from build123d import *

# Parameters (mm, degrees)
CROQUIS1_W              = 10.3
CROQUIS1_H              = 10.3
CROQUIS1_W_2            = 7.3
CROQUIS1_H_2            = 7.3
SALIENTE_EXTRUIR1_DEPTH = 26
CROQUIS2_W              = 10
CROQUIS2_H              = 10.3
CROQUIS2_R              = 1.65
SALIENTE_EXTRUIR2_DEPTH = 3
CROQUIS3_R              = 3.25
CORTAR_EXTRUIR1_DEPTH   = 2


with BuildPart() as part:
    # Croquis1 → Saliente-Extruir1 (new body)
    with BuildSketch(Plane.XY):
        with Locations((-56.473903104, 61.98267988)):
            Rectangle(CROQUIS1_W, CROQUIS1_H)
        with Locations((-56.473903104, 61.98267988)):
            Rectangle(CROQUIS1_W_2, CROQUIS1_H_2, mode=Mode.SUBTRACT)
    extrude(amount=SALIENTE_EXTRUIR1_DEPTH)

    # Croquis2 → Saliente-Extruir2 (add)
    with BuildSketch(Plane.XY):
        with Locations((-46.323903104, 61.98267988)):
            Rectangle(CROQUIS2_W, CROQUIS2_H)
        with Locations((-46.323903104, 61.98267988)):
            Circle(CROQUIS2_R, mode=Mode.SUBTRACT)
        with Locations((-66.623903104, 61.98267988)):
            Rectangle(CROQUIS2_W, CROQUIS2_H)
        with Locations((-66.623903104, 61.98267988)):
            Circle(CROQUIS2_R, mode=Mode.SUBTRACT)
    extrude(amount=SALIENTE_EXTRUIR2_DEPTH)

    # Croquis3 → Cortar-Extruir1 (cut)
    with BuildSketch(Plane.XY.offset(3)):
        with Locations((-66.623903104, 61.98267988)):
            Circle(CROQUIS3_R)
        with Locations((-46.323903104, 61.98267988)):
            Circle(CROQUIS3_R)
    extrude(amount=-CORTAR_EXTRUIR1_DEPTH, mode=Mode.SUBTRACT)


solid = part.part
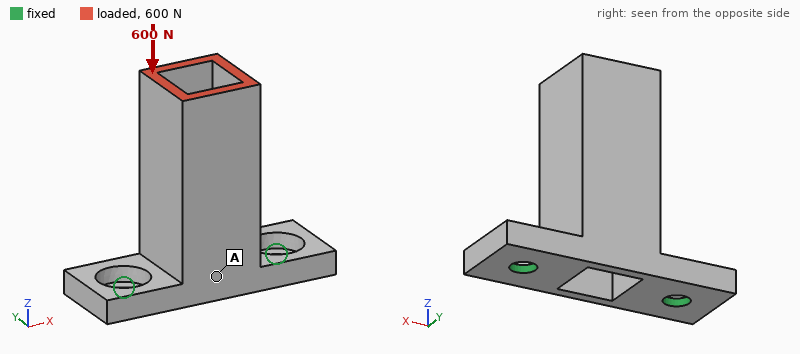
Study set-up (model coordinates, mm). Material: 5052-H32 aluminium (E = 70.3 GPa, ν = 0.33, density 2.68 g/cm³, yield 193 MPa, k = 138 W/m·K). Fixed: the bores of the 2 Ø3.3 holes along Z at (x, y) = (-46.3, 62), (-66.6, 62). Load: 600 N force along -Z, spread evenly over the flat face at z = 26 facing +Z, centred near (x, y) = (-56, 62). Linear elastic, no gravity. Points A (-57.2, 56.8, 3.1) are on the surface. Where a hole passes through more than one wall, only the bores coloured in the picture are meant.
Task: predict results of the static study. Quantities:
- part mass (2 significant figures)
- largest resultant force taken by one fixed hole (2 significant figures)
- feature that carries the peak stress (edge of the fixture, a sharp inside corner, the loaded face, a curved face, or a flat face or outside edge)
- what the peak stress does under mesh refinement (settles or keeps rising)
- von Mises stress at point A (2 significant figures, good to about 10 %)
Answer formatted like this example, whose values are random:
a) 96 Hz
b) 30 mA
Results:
a) 4.9 g
b) 410 N
c) edge of the fixture
d) keeps rising
e) 17 MPa
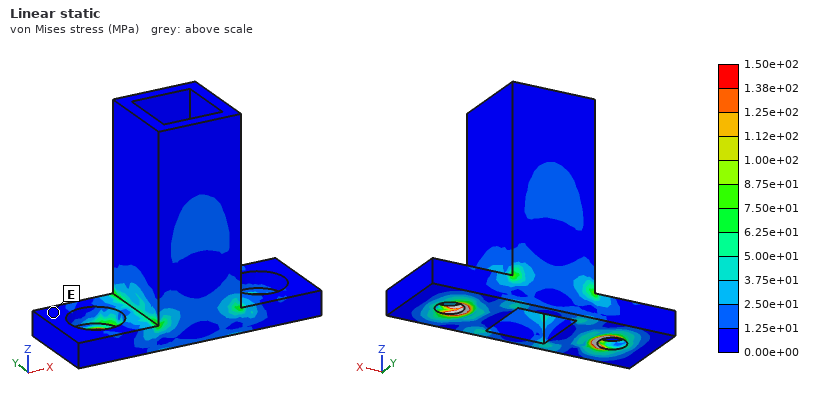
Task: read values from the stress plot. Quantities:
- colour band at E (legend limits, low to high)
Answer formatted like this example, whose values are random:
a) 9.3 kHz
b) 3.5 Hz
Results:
a) 0.00e+00 to 1.25e+01 MPa
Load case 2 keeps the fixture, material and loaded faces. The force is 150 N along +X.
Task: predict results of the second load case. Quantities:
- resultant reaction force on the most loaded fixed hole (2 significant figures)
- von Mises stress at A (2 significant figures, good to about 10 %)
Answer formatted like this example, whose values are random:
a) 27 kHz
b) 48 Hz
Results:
a) 240 N
b) 25 MPa
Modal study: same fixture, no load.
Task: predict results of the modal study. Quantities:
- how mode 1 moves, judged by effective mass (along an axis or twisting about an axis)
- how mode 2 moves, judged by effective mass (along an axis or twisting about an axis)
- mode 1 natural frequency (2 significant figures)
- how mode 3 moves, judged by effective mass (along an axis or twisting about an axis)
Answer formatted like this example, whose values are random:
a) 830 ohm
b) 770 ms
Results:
a) along Y
b) along X
c) 3000 Hz
d) along Z
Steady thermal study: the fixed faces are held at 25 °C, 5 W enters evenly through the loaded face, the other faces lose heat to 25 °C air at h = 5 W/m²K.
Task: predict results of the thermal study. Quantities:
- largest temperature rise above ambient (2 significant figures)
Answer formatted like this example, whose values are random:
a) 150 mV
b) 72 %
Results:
a) 22 K
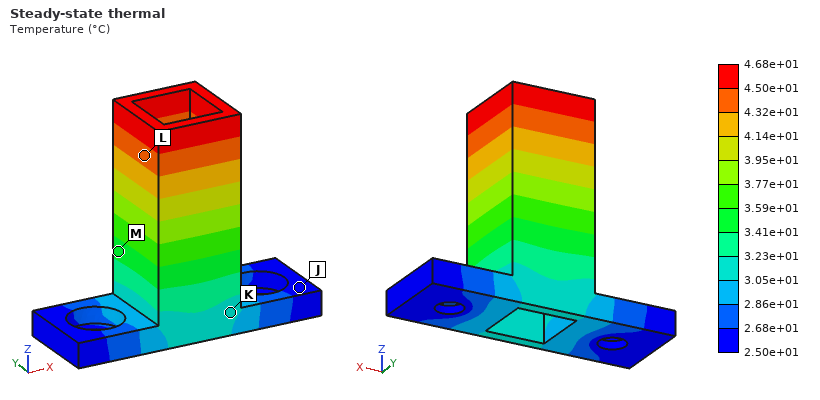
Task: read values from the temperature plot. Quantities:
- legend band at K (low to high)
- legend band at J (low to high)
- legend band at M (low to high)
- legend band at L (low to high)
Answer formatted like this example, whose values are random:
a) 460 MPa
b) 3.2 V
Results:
a) 3.05e+01 to 3.23e+01 °C
b) 2.50e+01 to 2.68e+01 °C
c) 3.41e+01 to 3.59e+01 °C
d) 4.32e+01 to 4.50e+01 °C
